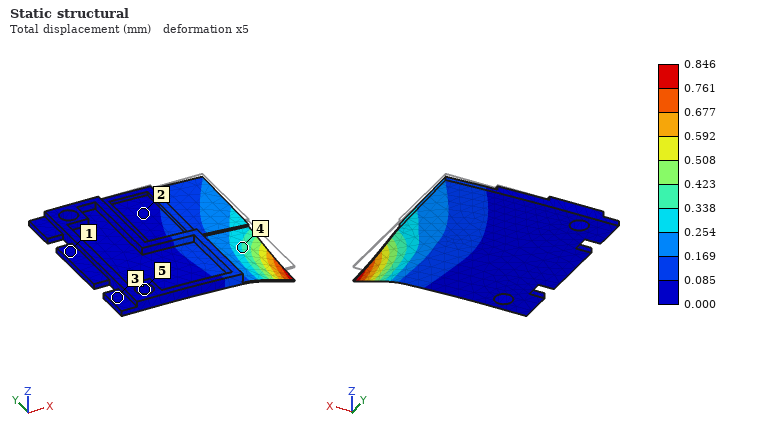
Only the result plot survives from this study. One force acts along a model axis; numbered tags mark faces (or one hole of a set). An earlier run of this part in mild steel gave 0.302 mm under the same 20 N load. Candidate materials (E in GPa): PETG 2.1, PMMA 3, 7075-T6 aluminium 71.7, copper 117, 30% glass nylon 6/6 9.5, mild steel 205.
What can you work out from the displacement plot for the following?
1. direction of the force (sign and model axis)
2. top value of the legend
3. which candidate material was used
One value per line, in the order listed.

-Z
0.846 mm
7075-T6 aluminium
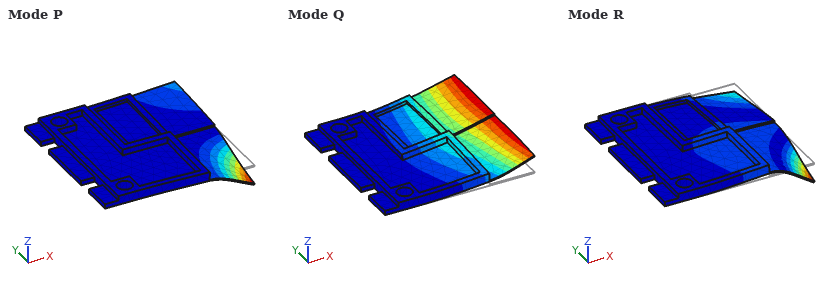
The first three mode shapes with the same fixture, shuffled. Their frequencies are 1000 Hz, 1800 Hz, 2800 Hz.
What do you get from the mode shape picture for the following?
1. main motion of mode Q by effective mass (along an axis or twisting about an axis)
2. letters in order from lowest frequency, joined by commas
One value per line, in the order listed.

along Z
Q, P, R
